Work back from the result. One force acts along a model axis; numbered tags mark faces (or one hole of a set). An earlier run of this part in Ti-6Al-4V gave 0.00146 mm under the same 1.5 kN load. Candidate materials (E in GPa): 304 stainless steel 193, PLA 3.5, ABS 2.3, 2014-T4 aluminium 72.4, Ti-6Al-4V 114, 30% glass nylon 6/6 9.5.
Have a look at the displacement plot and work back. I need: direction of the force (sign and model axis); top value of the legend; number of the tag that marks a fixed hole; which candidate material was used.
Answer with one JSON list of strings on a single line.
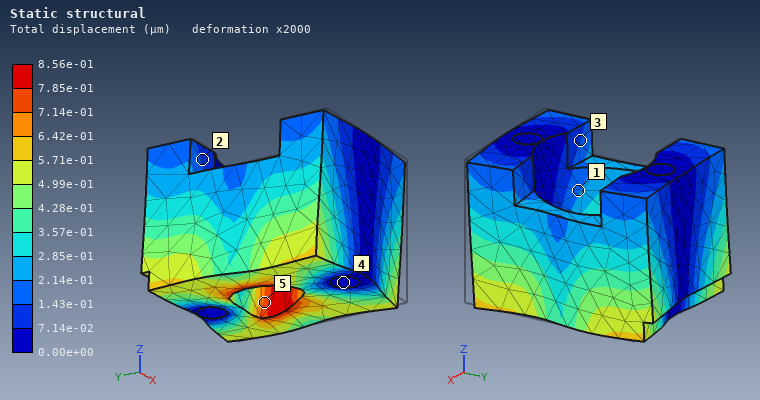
["+Y", "8.56e-01 µm", "4", "304 stainless steel"]
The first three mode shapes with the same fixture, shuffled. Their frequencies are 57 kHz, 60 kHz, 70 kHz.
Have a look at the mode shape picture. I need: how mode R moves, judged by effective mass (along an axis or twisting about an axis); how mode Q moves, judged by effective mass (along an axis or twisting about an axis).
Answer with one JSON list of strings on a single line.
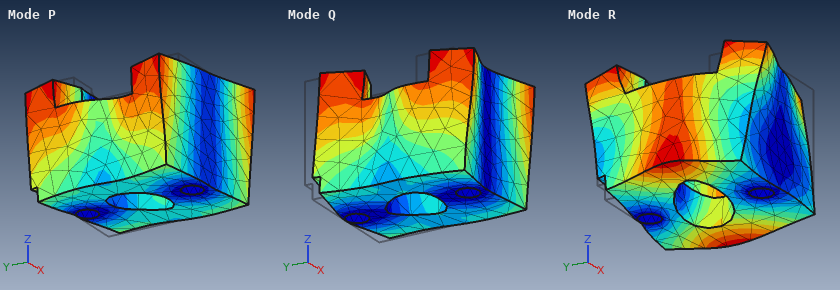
["twisting about Y", "along Y"]
